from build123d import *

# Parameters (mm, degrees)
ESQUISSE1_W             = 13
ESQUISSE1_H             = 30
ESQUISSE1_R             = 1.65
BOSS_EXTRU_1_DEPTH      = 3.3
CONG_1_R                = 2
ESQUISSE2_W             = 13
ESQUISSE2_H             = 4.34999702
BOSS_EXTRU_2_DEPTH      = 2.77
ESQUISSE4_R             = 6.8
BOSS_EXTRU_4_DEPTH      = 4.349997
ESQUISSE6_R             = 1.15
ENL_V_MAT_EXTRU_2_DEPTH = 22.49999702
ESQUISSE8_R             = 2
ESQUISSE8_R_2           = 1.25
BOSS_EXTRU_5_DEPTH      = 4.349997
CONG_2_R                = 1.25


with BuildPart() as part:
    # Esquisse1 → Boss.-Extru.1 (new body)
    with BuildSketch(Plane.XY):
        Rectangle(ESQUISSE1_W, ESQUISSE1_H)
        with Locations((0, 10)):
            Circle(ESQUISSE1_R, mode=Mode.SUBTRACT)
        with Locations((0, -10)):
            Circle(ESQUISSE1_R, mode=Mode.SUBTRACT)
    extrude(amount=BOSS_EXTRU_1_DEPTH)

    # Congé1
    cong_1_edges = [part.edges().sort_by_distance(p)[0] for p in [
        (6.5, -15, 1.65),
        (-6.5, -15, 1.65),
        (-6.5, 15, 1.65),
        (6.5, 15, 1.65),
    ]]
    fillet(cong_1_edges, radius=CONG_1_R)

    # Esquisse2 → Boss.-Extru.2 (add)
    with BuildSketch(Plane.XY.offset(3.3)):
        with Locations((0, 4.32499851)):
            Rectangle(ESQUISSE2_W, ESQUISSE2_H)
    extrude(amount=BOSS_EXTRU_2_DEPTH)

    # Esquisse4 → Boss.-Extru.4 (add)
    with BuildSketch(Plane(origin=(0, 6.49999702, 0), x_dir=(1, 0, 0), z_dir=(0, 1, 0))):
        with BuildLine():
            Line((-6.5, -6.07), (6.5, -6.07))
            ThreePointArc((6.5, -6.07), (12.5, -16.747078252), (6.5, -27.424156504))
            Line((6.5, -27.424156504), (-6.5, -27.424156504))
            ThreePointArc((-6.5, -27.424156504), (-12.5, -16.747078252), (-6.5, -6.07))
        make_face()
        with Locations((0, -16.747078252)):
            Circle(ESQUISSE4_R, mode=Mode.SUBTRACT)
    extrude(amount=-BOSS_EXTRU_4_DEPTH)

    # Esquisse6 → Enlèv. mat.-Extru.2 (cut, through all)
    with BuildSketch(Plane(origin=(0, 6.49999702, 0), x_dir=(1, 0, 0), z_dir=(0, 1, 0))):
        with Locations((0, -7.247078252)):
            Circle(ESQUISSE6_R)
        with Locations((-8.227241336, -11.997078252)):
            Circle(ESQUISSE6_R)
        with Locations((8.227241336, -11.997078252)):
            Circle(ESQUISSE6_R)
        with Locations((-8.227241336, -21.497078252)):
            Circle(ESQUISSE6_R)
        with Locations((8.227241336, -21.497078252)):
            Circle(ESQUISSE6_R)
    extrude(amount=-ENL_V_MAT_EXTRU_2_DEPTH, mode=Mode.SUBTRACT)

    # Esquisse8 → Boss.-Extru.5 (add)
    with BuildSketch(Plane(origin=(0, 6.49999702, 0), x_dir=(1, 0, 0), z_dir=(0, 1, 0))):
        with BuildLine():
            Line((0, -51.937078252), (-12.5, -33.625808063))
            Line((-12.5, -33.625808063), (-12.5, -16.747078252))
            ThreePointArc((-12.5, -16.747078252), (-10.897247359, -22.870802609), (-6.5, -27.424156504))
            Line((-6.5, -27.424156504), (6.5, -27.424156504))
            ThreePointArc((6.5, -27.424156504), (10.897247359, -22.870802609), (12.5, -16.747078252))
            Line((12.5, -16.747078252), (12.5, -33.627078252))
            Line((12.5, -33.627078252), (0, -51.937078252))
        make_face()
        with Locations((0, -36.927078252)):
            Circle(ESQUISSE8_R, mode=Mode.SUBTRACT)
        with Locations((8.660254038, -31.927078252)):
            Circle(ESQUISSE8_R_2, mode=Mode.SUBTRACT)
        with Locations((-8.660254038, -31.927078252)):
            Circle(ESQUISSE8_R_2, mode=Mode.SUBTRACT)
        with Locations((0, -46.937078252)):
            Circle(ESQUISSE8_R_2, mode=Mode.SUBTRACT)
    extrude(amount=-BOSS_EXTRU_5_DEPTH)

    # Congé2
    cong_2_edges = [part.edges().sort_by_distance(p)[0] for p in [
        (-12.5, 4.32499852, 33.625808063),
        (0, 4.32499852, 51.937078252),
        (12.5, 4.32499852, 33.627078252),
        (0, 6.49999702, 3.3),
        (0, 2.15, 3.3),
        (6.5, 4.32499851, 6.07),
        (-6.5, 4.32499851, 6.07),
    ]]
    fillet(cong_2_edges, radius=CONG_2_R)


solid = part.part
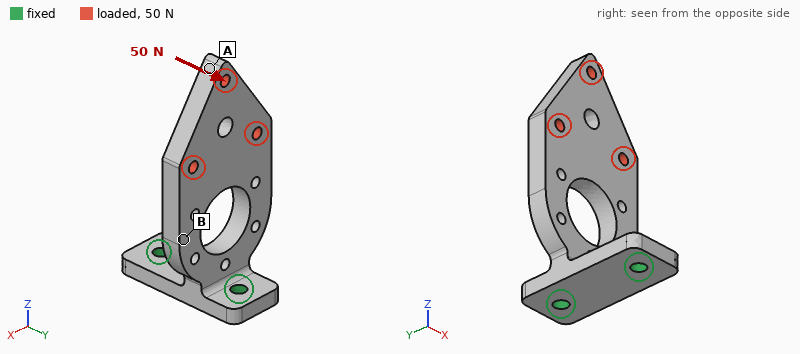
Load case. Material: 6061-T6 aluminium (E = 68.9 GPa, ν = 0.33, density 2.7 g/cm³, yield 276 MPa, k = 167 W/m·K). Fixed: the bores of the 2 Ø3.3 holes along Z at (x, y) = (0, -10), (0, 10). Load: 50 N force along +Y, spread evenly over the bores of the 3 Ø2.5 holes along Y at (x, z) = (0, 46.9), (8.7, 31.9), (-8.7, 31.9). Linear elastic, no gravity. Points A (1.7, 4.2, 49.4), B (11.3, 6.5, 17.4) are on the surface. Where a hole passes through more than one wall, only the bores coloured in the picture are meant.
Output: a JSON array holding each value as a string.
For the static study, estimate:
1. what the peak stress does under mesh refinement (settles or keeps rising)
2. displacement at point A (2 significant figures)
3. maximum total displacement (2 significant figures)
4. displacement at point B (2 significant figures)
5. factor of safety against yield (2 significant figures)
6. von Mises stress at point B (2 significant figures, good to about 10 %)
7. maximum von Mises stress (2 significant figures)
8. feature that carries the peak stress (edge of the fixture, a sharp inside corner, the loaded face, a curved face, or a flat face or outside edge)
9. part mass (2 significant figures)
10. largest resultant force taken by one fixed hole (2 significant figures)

["settles", "0.26 mm", "0.27 mm", "0.045 mm", "2.7", "26 MPa", "100 MPa", "a curved face", "12 g", "110 N"]
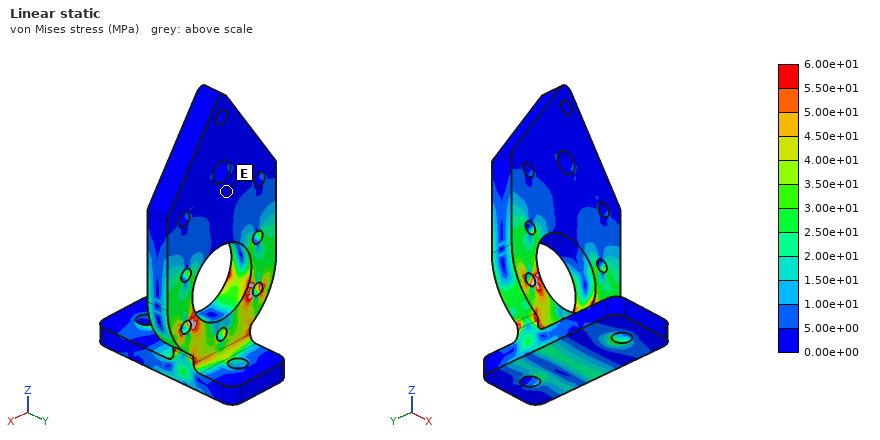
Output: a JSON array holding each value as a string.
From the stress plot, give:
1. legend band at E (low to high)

["0.00e+00 to 5.00e+00 MPa"]
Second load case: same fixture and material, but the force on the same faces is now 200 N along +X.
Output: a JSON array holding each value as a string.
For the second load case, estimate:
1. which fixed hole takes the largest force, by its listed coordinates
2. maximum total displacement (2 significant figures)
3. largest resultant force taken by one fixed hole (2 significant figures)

["(0, 10)", "0.31 mm", "180 N"]
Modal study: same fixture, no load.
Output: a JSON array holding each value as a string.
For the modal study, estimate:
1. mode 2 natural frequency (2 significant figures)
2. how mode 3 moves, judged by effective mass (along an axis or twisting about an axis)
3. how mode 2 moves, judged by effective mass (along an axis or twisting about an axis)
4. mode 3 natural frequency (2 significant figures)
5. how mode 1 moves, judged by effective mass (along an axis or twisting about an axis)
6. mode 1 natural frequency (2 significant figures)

["2100 Hz", "twisting about Z", "along X", "5200 Hz", "along Y", "1300 Hz"]
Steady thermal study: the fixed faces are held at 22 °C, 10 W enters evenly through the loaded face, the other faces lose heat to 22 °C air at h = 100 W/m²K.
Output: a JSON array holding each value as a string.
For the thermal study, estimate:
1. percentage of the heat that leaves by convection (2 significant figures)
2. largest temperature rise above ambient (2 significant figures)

["44 %", "30 K"]
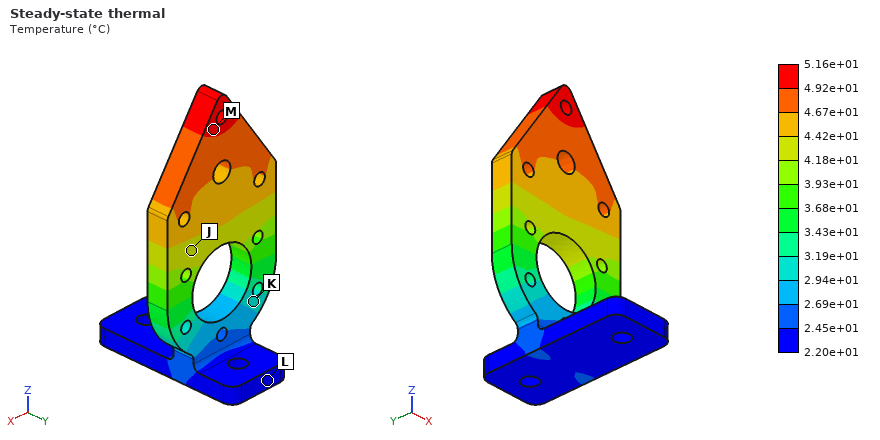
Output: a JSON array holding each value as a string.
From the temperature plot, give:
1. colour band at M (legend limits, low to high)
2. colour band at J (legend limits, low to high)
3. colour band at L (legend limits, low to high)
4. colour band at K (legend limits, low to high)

["4.92e+01 to 5.16e+01 °C", "4.18e+01 to 4.42e+01 °C", "2.20e+01 to 2.45e+01 °C", "2.94e+01 to 3.19e+01 °C"]
